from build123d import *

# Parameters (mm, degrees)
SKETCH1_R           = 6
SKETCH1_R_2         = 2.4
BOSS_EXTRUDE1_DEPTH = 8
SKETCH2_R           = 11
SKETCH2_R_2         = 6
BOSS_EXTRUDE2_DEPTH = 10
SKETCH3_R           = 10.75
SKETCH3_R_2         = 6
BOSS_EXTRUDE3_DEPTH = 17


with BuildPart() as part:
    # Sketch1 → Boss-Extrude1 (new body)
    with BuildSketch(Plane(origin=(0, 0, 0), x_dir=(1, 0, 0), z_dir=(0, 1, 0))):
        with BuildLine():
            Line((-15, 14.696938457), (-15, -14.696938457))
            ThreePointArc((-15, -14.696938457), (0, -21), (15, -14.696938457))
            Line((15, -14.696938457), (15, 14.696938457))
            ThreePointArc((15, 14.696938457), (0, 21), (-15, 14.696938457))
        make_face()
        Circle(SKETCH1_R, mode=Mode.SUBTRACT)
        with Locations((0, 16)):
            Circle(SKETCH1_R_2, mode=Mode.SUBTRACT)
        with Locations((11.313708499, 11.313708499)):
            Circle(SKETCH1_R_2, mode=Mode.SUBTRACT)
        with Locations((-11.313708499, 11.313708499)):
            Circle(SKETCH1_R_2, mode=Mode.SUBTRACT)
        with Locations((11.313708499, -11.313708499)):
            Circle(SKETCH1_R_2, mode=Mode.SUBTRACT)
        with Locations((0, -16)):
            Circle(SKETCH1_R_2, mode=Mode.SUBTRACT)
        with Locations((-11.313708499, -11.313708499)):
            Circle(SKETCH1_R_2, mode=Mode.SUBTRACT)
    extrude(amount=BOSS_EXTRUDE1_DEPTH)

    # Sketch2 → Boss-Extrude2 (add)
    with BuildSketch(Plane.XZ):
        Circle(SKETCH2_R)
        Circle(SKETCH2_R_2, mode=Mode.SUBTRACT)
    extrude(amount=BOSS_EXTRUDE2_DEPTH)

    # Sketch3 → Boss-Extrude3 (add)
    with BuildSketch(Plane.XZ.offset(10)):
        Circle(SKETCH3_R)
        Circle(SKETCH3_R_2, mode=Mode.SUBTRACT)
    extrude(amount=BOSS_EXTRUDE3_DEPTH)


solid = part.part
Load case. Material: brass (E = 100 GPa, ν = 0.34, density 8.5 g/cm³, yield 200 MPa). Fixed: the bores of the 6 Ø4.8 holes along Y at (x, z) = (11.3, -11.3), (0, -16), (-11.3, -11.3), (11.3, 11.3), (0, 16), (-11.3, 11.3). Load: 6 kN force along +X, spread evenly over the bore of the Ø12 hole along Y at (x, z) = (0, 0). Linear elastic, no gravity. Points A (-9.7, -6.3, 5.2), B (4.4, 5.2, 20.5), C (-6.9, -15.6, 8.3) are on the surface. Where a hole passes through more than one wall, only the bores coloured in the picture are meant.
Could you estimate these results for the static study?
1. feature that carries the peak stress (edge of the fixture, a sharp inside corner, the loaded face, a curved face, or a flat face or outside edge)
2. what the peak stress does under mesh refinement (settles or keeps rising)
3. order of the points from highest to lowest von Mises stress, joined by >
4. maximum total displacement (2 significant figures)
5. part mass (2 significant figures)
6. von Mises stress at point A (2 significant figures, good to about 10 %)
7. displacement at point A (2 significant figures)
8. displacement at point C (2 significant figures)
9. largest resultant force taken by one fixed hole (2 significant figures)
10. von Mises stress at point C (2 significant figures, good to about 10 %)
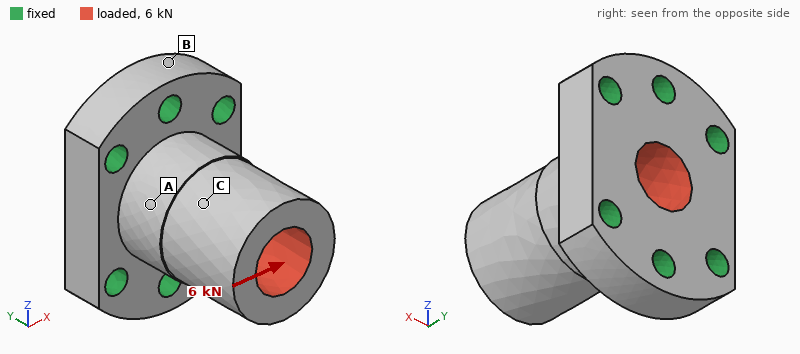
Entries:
edge of the fixture
keeps rising
A > C > B
39 µm
120 g
34 MPa
14 µm
24 µm
2.4 kN
18 MPa
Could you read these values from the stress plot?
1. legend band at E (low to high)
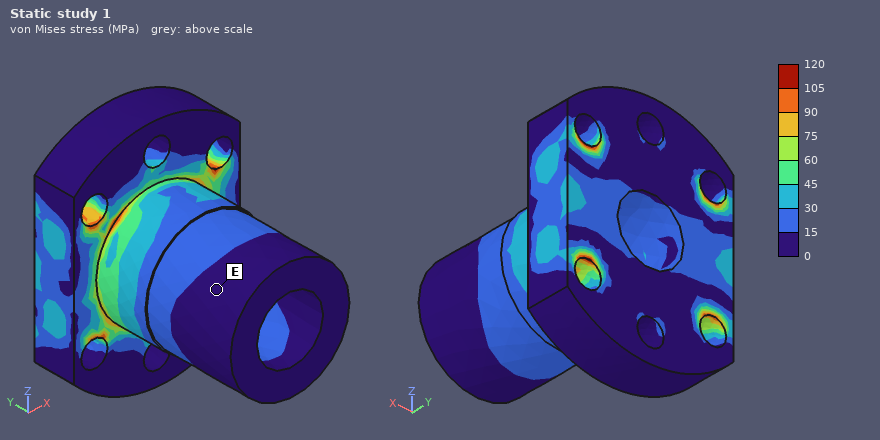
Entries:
0 to 15 MPa
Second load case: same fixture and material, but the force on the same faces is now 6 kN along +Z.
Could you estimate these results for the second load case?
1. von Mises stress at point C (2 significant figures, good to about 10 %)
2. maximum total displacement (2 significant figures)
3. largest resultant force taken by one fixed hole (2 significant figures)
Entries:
17 MPa
33 µm
2.0 kN
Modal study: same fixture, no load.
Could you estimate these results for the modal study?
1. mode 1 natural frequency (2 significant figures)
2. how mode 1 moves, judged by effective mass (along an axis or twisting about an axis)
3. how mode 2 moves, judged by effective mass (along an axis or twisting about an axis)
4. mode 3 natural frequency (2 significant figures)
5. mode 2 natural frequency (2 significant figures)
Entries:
8500 Hz
along X
along Z
18 kHz
9300 Hz
